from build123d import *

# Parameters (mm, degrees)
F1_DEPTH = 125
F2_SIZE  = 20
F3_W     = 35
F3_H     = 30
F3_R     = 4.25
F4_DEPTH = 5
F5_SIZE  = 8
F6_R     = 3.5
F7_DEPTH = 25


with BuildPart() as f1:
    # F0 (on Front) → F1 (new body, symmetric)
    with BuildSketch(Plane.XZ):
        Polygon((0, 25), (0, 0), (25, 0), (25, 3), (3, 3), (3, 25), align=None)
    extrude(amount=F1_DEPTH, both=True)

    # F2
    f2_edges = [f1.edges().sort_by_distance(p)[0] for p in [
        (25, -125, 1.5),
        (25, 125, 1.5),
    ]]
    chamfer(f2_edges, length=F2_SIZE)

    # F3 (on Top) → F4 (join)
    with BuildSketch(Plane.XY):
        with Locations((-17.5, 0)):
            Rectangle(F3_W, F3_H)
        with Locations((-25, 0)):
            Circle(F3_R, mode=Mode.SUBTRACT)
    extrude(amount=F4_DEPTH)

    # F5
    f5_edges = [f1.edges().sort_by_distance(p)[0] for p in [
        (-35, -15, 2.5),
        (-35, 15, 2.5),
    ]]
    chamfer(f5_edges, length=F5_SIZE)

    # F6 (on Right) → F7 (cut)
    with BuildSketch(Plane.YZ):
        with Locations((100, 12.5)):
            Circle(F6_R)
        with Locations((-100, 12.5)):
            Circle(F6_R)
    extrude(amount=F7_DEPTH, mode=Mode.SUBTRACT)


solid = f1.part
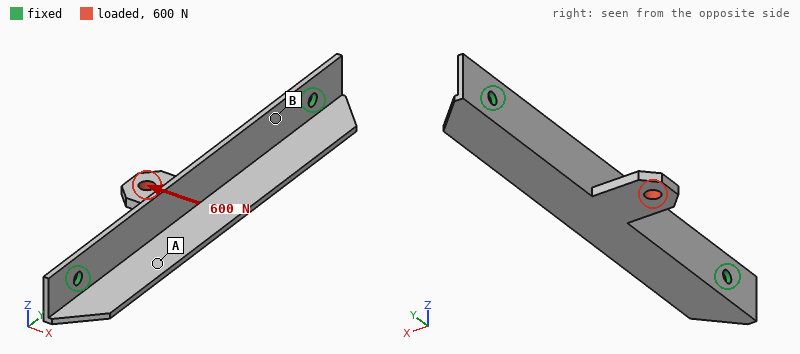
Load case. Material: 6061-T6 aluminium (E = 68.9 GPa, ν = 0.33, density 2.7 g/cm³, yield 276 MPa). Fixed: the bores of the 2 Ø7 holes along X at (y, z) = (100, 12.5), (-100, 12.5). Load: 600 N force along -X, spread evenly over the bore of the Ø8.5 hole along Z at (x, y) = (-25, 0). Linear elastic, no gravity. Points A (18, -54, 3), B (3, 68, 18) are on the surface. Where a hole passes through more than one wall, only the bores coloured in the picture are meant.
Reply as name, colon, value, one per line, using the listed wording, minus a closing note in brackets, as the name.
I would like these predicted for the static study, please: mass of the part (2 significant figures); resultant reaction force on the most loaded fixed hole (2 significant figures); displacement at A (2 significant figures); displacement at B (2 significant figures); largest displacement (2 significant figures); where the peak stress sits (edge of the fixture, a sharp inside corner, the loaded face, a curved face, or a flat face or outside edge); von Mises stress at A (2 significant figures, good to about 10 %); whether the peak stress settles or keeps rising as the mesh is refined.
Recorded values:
mass of the part: 100 g
resultant reaction force on the most loaded fixed hole: 690 N
displacement at A: 0.13 mm
displacement at B: 0.054 mm
largest displacement: 0.19 mm
where the peak stress sits: edge of the fixture
von Mises stress at A: 18 MPa
whether the peak stress settles or keeps rising as the mesh is refined: keeps rising
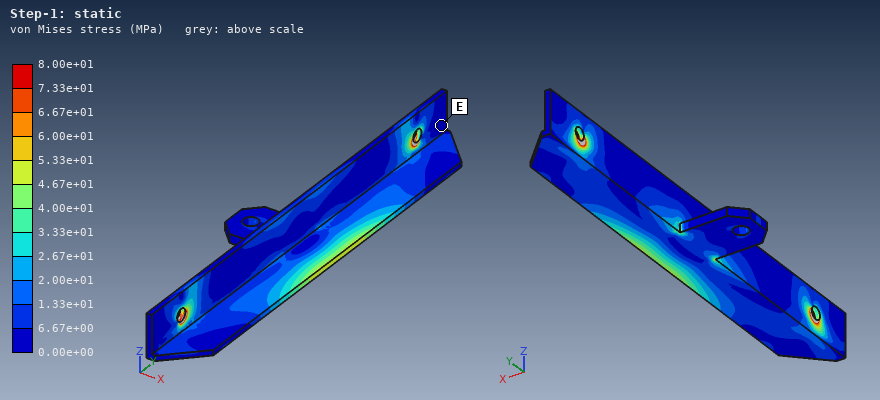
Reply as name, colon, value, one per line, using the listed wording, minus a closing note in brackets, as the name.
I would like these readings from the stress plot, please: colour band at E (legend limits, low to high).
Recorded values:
colour band at E: 0.00e+00 to 6.67e+00 MPa
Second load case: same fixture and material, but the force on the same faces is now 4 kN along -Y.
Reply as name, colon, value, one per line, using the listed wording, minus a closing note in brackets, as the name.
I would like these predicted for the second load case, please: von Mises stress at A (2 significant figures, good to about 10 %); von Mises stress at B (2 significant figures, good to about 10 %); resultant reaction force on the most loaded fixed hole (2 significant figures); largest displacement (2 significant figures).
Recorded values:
von Mises stress at A: 43 MPa
von Mises stress at B: 22 MPa
resultant reaction force on the most loaded fixed hole: 2.1 kN
largest displacement: 0.43 mm
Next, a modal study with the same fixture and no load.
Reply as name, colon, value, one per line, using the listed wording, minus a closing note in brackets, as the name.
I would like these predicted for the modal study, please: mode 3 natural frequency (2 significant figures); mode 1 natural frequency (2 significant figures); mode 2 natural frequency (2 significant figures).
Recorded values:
mode 3 natural frequency: 1800 Hz
mode 1 natural frequency: 750 Hz
mode 2 natural frequency: 1200 Hz
